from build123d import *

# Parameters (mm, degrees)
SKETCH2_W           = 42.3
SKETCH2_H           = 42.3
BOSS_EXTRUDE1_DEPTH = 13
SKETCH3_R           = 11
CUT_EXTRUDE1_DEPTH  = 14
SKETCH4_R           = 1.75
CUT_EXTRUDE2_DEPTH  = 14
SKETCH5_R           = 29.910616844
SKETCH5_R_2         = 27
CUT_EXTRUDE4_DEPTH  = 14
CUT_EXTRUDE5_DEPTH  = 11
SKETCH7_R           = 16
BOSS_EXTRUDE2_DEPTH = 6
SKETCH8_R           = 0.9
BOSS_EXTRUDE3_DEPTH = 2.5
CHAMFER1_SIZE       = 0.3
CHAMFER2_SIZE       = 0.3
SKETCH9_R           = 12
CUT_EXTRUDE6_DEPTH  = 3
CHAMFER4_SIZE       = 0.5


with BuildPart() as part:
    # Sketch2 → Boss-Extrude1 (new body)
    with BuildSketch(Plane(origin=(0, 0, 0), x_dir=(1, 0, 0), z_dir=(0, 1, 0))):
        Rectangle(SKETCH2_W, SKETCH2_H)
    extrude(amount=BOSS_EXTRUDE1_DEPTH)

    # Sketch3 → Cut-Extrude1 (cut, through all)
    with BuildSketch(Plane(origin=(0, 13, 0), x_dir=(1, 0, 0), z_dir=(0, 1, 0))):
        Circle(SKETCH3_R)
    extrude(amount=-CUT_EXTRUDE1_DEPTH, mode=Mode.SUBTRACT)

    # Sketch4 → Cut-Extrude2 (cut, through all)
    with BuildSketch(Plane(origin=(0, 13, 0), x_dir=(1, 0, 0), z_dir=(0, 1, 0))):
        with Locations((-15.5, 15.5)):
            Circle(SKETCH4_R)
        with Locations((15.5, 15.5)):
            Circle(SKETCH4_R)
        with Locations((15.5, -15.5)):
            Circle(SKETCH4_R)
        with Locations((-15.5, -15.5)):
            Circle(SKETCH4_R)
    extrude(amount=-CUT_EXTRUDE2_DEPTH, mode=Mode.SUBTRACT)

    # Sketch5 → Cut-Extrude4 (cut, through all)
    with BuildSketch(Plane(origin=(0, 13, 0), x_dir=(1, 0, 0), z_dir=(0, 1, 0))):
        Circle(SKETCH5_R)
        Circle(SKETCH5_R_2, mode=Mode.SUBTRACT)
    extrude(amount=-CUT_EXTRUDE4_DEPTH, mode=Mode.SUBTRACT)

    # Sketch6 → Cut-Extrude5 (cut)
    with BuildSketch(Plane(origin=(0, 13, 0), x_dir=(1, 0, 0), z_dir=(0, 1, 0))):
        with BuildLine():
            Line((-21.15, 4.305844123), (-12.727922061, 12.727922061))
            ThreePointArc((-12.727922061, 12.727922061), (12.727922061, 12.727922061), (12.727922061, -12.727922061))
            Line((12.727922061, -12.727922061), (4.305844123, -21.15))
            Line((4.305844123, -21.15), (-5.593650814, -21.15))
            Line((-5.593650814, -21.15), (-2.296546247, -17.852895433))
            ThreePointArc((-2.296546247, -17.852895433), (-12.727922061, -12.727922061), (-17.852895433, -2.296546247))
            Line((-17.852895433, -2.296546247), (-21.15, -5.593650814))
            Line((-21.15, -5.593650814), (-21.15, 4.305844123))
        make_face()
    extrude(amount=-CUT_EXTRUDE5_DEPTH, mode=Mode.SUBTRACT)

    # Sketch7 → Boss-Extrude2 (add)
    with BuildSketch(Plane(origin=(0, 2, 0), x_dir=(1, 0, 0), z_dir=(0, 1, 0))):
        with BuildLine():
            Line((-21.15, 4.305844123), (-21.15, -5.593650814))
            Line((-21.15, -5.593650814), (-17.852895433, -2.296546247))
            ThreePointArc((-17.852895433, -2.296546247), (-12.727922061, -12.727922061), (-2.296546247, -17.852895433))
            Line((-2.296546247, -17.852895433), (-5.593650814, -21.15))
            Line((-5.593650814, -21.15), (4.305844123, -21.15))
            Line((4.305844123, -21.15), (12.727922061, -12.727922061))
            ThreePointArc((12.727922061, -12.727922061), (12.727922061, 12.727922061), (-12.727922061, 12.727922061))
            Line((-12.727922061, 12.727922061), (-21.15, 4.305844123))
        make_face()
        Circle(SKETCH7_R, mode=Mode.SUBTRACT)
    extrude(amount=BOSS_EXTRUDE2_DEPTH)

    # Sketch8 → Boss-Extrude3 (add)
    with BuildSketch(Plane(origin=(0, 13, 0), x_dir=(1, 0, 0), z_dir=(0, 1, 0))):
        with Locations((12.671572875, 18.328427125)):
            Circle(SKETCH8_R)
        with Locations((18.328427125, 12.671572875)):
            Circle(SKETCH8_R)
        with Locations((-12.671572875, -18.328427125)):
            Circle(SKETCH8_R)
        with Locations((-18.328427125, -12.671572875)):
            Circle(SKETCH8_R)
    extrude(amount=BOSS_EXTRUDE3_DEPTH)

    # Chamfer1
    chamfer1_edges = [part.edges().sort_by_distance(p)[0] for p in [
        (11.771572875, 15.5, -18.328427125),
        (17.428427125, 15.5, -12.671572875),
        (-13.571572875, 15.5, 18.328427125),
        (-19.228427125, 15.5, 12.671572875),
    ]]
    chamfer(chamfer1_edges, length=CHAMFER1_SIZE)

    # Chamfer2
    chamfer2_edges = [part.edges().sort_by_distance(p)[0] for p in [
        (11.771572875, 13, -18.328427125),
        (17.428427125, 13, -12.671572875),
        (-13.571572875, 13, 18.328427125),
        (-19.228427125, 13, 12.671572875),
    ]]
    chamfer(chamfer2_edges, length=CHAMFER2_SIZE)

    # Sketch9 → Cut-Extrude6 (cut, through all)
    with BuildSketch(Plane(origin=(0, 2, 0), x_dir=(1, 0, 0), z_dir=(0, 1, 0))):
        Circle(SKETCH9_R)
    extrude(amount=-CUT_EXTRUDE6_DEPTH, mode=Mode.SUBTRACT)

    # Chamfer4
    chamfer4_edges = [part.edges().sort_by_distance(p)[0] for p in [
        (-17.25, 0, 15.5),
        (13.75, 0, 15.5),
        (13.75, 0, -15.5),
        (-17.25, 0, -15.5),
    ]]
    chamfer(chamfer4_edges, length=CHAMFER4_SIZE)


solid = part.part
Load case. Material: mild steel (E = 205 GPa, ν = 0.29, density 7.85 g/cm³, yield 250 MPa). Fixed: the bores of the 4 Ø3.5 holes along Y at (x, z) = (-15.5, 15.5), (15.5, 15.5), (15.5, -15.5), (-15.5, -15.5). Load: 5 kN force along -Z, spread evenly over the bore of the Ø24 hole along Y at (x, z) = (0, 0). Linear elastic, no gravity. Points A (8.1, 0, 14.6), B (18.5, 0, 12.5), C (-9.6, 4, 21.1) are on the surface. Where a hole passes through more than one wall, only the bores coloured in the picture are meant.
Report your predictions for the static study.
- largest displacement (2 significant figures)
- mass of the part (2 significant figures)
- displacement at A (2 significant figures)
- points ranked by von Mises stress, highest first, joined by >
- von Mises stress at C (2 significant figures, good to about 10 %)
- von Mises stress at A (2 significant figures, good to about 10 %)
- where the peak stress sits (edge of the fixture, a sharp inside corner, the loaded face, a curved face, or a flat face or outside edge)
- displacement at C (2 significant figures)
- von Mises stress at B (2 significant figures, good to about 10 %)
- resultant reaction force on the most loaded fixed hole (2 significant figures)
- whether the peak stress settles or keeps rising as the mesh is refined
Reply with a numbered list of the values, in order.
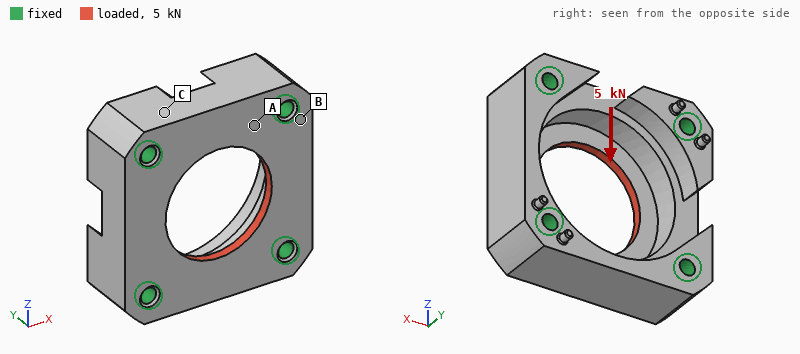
1. 5.0 µm
2. 87 g
3. 2.2 µm
4. A > C > B
5. 18 MPa
6. 43 MPa
7. edge of the fixture
8. 1.3 µm
9. 6.3 MPa
10. 1.3 kN
11. keeps rising
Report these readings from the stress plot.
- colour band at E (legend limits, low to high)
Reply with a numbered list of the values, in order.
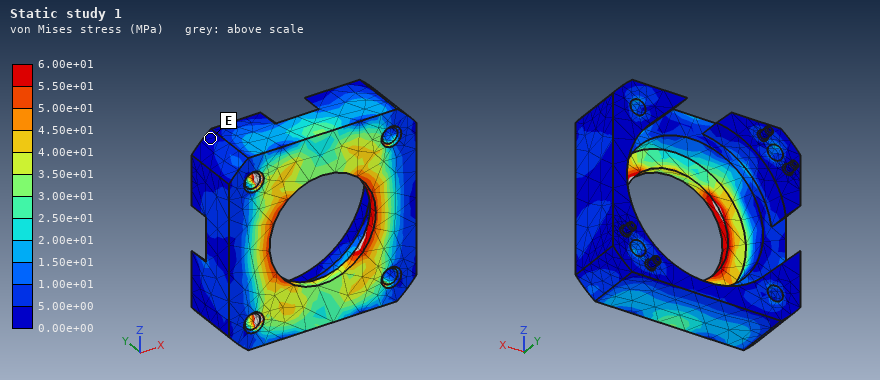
1. 0.00e+00 to 5.00e+00 MPa
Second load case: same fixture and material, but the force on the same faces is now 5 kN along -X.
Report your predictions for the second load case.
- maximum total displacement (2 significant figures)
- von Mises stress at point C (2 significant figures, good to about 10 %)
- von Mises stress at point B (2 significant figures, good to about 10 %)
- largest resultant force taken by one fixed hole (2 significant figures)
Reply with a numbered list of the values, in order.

1. 5.0 µm
2. 7.1 MPa
3. 25 MPa
4. 1.3 kN
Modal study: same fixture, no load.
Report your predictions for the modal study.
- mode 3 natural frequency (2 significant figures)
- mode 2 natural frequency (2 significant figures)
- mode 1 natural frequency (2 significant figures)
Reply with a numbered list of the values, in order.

1. 40 kHz
2. 40 kHz
3. 32 kHz
